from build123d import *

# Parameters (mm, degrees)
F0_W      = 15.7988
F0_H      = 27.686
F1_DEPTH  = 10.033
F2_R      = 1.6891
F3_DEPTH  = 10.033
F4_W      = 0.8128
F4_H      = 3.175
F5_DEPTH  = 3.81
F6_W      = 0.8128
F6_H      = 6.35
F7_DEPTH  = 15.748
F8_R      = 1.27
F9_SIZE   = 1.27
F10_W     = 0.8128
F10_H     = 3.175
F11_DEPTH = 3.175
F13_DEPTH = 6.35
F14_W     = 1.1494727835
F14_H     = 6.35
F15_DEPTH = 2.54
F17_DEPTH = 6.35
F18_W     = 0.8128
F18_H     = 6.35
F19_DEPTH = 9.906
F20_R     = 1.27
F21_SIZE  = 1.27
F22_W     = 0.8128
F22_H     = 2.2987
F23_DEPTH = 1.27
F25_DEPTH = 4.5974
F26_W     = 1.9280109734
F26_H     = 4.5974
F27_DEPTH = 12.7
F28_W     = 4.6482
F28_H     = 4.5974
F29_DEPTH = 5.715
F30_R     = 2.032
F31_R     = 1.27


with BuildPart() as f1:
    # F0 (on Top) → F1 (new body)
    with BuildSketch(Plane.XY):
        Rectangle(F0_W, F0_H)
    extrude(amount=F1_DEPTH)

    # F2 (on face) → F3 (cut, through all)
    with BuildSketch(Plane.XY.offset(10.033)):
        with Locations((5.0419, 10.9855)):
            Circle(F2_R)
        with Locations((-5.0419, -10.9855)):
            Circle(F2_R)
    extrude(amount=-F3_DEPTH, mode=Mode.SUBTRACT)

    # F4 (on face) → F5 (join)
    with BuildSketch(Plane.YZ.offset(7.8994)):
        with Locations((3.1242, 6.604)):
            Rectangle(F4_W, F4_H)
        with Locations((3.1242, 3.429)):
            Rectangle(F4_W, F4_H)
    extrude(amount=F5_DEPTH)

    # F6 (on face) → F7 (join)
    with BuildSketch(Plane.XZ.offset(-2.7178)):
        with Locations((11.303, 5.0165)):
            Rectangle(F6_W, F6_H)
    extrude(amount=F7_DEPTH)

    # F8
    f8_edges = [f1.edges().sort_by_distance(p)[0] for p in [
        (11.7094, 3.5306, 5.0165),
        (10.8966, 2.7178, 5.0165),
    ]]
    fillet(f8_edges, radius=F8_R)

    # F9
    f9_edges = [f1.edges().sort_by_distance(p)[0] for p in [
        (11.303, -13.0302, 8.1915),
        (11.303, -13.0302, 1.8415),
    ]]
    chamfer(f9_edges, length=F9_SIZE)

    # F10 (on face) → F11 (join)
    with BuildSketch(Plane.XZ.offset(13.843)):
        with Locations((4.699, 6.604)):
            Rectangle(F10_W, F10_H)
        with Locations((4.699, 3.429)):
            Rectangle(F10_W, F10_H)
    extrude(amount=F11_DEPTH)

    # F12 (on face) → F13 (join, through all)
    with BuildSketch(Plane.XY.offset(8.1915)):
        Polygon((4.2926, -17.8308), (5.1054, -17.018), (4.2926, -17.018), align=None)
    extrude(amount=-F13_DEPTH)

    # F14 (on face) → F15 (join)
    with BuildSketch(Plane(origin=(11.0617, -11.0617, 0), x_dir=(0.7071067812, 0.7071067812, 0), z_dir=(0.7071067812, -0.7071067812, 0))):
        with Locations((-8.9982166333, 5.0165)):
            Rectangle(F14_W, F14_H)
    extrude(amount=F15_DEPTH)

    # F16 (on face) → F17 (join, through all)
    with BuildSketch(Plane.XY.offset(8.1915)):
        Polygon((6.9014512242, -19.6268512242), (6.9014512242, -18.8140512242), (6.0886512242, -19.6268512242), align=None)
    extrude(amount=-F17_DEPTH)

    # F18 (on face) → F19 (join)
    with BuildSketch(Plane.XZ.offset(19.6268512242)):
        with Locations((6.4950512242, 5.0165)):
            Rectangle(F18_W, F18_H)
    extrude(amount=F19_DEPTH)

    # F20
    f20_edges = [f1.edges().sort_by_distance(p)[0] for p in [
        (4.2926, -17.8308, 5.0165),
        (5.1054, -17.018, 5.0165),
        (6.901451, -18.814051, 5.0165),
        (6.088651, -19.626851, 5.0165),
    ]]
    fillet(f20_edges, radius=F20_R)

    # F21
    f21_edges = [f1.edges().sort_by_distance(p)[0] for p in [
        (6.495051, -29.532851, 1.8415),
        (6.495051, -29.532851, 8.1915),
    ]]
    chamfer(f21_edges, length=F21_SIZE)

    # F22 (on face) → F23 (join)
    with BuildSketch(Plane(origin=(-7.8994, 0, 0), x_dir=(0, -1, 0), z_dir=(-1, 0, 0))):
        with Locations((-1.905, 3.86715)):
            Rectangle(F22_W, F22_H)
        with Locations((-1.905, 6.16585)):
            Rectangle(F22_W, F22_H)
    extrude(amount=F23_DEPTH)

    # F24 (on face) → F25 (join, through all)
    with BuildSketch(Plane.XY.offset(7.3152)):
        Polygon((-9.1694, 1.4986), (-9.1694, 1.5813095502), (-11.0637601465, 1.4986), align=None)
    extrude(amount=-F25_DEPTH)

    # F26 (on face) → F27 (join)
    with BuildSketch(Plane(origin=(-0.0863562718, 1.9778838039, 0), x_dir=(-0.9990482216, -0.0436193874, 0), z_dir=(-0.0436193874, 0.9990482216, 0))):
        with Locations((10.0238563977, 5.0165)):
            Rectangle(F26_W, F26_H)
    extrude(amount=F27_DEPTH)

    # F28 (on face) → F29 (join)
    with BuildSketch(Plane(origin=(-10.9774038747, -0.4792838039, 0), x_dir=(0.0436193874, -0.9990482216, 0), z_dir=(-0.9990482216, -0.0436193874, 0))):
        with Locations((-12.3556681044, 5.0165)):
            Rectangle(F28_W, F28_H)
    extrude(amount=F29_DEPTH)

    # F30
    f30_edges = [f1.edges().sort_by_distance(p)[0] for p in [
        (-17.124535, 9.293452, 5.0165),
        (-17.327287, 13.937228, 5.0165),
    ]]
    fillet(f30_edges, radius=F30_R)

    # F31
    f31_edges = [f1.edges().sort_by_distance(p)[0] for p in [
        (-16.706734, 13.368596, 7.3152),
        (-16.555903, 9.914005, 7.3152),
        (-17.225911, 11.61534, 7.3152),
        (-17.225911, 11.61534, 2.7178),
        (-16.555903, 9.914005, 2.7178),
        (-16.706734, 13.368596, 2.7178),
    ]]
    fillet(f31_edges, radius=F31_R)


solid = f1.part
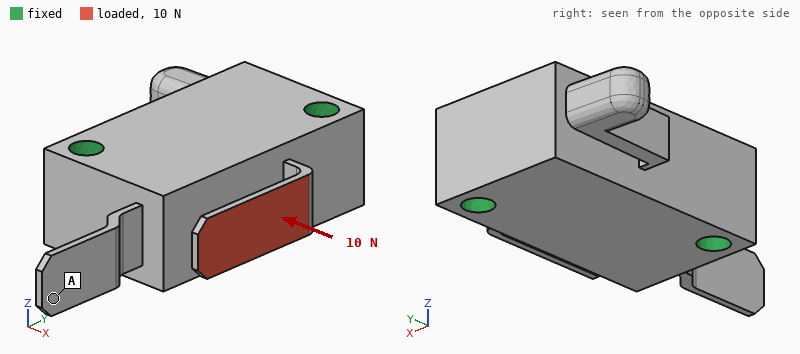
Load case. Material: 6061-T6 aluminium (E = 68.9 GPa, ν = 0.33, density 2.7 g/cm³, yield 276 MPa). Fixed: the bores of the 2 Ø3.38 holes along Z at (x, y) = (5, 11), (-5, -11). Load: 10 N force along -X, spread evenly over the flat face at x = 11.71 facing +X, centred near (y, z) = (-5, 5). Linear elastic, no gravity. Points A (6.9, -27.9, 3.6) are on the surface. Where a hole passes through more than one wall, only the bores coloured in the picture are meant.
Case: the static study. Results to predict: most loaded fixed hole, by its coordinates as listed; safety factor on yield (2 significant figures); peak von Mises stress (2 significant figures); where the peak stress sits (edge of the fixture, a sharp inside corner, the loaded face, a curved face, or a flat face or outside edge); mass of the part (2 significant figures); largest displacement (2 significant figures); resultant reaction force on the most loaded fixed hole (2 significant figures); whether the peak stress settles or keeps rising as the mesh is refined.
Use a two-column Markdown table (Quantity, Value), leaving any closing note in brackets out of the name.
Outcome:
| Quantity | Value |
|---|---|
| most loaded fixed hole, by its coordinates as listed | (-5, -11) |
| safety factor on yield | 2.2 |
| peak von Mises stress | 120 MPa |
| where the peak stress sits | a flat face or outside edge |
| mass of the part | 12 g |
| largest displacement | 0.40 mm |
| resultant reaction force on the most loaded fixed hole | 7.8 N |
| whether the peak stress settles or keeps rising as the mesh is refined | settles |
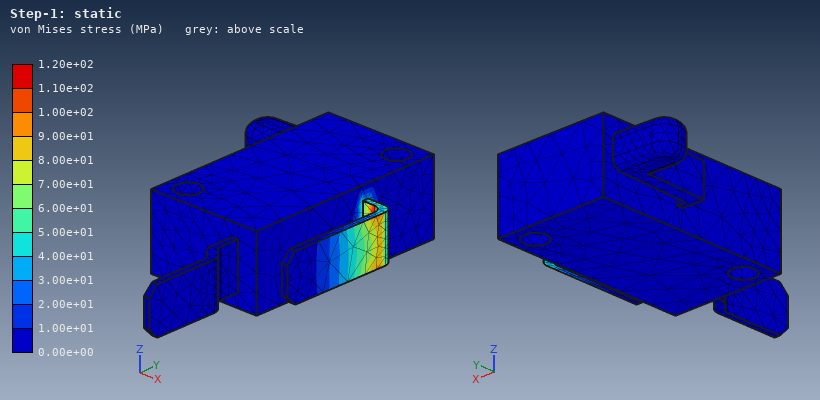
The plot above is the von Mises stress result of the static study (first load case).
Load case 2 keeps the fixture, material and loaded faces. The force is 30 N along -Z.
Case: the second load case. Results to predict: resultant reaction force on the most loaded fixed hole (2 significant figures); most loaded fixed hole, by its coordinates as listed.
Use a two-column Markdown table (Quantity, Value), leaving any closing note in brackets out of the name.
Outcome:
| Quantity | Value |
|---|---|
| resultant reaction force on the most loaded fixed hole | 18 N |
| most loaded fixed hole, by its coordinates as listed | (5, 11) |
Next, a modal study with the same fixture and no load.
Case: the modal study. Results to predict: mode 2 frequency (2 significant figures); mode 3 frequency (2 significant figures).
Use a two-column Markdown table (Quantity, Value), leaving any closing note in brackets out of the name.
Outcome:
| Quantity | Value |
|---|---|
| mode 2 frequency | 2200 Hz |
| mode 3 frequency | 2900 Hz |
